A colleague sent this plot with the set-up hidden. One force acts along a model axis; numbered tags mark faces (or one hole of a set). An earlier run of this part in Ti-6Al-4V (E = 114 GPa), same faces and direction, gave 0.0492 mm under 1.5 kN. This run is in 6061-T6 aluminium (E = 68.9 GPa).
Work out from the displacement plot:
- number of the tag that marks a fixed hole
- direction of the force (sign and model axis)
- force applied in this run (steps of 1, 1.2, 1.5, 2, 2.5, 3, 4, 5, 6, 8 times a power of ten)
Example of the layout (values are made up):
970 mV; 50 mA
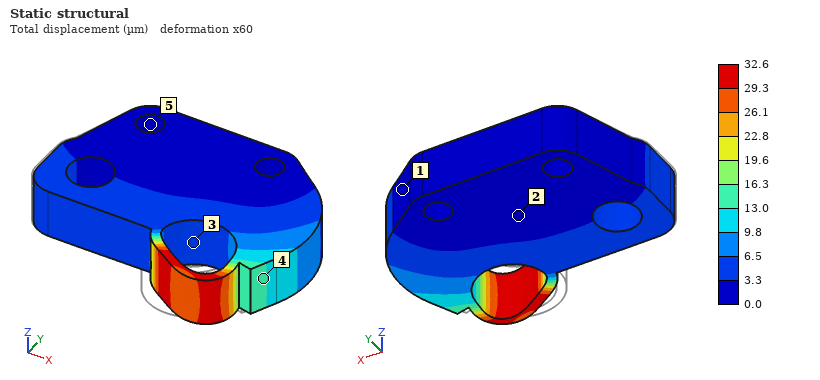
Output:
5; +X; 600 N
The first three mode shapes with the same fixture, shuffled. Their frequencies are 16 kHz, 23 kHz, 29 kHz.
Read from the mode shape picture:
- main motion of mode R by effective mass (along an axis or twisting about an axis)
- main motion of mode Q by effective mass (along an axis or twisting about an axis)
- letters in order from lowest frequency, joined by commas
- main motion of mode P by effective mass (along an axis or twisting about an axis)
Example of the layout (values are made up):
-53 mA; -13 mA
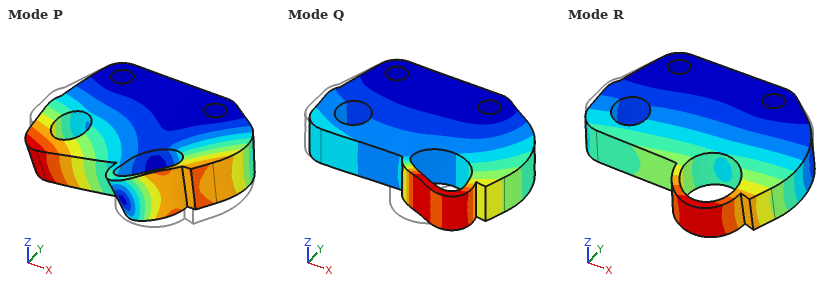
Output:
along Z; along X; R, P, Q; twisting about Y
